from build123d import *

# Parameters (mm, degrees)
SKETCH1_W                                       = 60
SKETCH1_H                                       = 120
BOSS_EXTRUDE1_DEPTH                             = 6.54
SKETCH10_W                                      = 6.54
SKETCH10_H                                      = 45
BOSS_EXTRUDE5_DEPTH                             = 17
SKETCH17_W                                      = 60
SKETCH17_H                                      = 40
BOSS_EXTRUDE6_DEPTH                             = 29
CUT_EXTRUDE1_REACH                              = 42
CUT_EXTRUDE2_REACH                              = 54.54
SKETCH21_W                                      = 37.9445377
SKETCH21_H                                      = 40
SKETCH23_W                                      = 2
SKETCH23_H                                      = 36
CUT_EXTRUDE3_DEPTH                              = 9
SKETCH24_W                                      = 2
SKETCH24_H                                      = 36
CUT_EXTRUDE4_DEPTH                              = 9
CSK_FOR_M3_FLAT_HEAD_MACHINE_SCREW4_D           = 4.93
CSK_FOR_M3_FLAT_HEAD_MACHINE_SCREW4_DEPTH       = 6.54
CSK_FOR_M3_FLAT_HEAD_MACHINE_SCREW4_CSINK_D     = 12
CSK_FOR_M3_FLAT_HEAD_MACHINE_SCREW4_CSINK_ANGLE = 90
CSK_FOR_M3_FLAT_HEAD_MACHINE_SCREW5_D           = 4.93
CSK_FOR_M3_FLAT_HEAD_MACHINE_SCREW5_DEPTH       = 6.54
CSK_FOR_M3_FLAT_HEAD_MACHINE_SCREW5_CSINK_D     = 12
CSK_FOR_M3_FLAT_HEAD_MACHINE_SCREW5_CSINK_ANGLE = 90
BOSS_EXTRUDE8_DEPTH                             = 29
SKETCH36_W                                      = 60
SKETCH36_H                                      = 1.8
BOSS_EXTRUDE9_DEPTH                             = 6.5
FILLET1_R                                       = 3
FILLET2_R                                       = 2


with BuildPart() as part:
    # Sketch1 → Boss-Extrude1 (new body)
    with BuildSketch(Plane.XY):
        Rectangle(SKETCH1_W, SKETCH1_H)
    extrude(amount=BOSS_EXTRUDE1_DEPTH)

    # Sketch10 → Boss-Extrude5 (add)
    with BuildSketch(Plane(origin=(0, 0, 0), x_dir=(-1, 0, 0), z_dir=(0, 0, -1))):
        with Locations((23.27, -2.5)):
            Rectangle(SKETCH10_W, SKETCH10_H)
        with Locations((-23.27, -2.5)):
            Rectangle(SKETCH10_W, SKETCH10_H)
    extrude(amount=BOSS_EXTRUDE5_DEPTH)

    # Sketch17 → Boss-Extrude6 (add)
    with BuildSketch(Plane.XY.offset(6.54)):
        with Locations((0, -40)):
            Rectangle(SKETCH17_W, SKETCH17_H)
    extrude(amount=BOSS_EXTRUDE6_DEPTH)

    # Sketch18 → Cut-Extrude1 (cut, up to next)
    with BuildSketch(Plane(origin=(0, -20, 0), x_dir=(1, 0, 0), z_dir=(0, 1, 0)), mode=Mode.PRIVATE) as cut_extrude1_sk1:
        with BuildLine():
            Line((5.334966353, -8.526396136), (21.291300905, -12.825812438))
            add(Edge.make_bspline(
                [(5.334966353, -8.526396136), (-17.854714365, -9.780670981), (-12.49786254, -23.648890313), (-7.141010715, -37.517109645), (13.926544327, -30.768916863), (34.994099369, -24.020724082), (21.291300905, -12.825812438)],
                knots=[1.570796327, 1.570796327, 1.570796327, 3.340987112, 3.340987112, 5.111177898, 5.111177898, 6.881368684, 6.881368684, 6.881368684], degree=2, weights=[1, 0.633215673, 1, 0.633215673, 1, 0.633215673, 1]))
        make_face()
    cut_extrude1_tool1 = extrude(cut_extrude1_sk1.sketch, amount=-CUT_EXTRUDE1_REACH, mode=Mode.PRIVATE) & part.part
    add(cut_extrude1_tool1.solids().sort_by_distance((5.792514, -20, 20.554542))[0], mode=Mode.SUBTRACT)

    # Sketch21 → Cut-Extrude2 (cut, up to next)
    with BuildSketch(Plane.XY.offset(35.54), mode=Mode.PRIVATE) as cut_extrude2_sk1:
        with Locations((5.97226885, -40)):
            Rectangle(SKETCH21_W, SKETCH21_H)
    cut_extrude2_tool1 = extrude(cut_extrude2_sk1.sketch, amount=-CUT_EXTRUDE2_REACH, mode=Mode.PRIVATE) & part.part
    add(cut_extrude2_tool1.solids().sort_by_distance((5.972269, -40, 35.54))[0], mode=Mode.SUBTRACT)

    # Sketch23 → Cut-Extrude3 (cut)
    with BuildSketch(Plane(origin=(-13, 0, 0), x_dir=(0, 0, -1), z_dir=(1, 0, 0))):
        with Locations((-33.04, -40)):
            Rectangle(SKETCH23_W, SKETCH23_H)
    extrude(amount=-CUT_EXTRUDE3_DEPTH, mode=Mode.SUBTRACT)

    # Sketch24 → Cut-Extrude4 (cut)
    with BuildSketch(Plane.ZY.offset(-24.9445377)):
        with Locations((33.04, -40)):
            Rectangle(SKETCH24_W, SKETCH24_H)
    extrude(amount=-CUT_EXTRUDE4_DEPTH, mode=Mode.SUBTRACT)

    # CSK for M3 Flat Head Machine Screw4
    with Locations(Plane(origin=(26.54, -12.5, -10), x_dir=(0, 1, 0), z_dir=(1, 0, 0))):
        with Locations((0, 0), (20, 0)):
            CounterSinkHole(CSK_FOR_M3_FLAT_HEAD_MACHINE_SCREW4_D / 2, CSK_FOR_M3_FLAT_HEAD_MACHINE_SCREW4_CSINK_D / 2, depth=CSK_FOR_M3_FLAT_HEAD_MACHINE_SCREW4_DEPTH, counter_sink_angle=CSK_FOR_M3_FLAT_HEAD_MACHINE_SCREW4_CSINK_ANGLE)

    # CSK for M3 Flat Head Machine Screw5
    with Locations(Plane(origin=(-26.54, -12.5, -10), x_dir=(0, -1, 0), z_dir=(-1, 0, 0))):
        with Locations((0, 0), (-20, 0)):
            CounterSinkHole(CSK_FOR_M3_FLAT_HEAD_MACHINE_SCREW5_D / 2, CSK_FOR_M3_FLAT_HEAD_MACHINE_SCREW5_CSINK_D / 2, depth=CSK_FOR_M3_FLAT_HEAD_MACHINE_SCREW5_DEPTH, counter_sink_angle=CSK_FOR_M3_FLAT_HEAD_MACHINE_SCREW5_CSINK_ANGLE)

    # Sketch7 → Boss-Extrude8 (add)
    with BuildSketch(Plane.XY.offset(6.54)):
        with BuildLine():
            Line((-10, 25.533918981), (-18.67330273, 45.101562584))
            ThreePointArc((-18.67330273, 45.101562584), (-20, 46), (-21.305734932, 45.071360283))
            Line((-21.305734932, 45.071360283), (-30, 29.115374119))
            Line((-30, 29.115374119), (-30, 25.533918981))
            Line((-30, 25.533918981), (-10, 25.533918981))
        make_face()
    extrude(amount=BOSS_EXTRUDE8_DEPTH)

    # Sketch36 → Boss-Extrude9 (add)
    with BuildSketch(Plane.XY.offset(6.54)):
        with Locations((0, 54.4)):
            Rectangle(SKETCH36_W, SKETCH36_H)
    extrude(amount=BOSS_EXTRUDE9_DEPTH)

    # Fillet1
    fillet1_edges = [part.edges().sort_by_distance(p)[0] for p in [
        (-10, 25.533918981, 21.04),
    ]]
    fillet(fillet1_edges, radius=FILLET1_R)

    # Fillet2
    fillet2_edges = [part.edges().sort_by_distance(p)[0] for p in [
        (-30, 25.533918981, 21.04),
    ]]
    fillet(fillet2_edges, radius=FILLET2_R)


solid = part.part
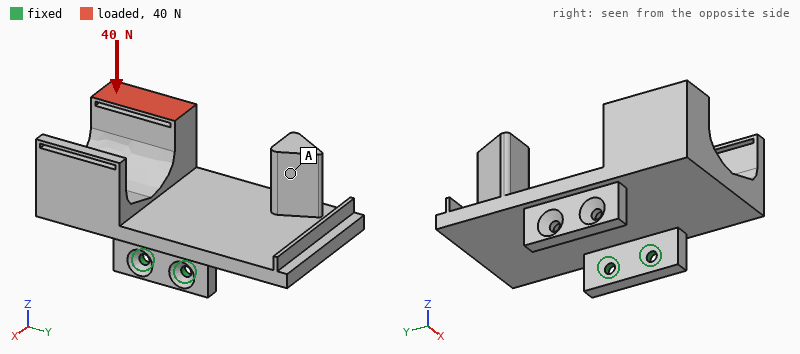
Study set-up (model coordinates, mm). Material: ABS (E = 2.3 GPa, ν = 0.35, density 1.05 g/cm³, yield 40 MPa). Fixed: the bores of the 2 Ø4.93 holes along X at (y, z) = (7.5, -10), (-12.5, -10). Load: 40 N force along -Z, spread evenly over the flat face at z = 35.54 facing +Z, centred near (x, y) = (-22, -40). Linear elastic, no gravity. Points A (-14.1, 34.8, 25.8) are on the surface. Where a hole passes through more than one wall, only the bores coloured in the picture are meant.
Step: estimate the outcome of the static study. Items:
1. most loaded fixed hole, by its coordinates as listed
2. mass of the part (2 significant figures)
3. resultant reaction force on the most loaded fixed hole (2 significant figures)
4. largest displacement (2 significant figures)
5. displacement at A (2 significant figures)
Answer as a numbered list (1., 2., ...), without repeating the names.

1. (-12.5, -10)
2. 100 g
3. 85 N
4. 1.6 mm
5. 0.73 mm
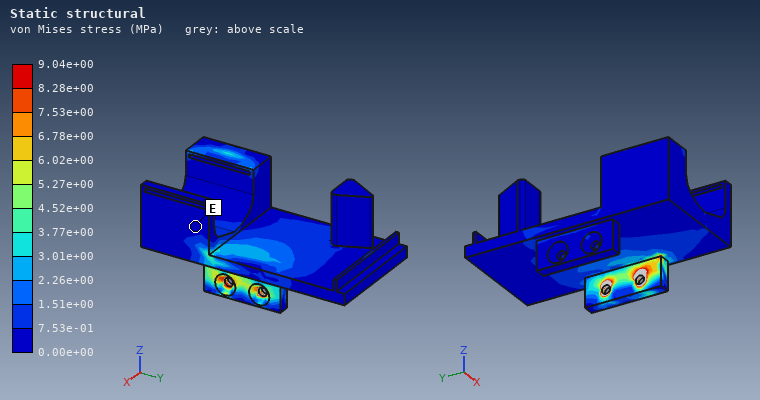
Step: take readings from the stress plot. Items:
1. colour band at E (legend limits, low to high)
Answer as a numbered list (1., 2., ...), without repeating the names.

1. 0.00e+00 to 7.53e-01 MPa
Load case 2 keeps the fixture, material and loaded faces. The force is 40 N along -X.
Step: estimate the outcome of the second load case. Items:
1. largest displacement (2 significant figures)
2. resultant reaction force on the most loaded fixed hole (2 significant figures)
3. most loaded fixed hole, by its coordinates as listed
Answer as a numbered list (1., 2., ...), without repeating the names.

1. 1.5 mm
2. 83 N
3. (-12.5, -10)
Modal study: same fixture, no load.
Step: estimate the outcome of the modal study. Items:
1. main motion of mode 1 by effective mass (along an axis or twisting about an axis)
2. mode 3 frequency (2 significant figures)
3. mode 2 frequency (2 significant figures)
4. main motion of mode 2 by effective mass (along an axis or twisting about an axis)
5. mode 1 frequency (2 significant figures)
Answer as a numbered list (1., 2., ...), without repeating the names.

1. along Z
2. 290 Hz
3. 240 Hz
4. along Y
5. 130 Hz
